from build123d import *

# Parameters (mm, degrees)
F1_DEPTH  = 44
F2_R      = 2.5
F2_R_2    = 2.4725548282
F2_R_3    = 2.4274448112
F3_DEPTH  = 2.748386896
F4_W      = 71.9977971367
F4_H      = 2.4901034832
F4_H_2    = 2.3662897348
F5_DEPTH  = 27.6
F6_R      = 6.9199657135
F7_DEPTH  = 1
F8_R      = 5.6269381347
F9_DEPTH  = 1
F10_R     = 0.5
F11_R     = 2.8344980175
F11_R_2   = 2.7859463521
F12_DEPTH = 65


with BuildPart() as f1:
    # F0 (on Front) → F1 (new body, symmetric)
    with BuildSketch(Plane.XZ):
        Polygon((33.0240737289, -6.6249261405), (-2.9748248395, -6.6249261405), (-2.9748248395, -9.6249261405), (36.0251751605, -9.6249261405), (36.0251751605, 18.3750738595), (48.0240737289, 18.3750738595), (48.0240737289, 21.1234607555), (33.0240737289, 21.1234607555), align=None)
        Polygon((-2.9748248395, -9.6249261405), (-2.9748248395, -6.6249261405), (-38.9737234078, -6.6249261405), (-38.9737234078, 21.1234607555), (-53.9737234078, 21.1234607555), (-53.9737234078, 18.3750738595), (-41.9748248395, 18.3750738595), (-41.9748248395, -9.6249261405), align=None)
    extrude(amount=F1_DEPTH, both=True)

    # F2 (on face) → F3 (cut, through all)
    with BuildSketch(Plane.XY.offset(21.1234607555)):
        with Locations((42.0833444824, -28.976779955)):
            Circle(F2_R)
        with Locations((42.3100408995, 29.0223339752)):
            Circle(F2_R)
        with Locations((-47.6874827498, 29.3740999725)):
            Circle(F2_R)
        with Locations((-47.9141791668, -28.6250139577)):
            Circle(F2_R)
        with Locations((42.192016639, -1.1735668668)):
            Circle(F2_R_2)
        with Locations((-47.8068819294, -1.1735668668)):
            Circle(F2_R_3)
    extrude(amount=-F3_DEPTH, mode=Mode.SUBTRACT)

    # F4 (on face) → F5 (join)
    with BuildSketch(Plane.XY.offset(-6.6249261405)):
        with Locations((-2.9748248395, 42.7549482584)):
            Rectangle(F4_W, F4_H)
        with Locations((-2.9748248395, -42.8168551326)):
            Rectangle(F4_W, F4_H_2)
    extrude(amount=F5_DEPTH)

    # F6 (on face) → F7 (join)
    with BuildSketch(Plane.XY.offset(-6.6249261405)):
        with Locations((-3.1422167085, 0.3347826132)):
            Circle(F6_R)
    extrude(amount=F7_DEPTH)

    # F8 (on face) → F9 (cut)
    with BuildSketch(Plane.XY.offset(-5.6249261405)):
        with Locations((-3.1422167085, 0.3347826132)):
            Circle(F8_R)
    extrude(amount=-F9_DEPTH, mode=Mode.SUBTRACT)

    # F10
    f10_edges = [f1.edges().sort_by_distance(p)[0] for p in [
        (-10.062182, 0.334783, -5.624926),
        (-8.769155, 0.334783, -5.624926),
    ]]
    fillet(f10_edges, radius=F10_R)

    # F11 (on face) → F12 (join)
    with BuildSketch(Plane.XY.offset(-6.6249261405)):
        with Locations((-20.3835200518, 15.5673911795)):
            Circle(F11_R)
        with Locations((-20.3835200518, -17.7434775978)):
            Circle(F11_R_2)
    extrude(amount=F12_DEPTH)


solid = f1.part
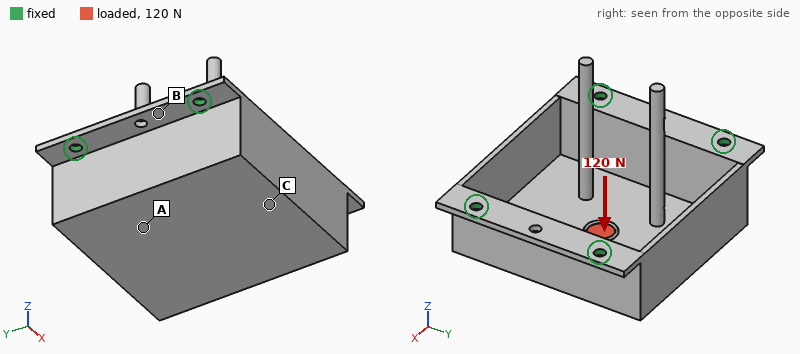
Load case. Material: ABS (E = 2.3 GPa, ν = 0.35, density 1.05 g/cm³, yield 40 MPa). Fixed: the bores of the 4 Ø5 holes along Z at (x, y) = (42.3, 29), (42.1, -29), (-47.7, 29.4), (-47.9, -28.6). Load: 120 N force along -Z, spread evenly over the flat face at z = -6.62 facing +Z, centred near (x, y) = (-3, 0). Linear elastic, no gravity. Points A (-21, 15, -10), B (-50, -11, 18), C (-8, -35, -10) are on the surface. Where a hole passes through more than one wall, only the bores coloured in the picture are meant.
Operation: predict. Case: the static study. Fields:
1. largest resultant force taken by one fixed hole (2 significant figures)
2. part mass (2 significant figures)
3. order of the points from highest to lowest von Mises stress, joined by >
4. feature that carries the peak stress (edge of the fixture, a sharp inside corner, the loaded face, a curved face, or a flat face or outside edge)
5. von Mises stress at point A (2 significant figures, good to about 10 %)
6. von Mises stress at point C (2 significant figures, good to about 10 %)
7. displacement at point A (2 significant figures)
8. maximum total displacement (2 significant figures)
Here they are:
36 N
56 g
A > C > B
a flat face or outside edge
4.0 MPa
2.4 MPa
0.40 mm
1.8 mm
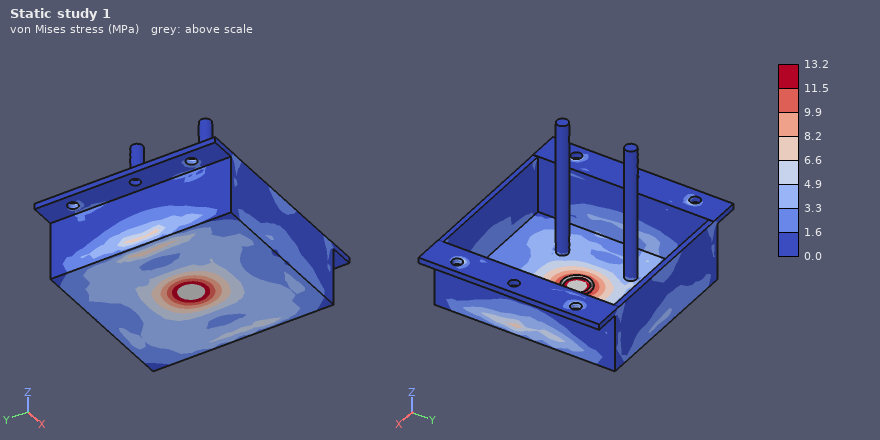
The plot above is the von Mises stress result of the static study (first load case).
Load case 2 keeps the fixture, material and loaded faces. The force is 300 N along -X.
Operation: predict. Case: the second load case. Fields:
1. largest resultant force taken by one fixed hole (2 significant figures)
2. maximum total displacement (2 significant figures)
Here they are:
110 N
0.23 mm
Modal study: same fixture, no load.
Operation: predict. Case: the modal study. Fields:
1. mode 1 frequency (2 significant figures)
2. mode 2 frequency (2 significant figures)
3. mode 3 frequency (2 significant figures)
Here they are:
240 Hz
240 Hz
250 Hz
